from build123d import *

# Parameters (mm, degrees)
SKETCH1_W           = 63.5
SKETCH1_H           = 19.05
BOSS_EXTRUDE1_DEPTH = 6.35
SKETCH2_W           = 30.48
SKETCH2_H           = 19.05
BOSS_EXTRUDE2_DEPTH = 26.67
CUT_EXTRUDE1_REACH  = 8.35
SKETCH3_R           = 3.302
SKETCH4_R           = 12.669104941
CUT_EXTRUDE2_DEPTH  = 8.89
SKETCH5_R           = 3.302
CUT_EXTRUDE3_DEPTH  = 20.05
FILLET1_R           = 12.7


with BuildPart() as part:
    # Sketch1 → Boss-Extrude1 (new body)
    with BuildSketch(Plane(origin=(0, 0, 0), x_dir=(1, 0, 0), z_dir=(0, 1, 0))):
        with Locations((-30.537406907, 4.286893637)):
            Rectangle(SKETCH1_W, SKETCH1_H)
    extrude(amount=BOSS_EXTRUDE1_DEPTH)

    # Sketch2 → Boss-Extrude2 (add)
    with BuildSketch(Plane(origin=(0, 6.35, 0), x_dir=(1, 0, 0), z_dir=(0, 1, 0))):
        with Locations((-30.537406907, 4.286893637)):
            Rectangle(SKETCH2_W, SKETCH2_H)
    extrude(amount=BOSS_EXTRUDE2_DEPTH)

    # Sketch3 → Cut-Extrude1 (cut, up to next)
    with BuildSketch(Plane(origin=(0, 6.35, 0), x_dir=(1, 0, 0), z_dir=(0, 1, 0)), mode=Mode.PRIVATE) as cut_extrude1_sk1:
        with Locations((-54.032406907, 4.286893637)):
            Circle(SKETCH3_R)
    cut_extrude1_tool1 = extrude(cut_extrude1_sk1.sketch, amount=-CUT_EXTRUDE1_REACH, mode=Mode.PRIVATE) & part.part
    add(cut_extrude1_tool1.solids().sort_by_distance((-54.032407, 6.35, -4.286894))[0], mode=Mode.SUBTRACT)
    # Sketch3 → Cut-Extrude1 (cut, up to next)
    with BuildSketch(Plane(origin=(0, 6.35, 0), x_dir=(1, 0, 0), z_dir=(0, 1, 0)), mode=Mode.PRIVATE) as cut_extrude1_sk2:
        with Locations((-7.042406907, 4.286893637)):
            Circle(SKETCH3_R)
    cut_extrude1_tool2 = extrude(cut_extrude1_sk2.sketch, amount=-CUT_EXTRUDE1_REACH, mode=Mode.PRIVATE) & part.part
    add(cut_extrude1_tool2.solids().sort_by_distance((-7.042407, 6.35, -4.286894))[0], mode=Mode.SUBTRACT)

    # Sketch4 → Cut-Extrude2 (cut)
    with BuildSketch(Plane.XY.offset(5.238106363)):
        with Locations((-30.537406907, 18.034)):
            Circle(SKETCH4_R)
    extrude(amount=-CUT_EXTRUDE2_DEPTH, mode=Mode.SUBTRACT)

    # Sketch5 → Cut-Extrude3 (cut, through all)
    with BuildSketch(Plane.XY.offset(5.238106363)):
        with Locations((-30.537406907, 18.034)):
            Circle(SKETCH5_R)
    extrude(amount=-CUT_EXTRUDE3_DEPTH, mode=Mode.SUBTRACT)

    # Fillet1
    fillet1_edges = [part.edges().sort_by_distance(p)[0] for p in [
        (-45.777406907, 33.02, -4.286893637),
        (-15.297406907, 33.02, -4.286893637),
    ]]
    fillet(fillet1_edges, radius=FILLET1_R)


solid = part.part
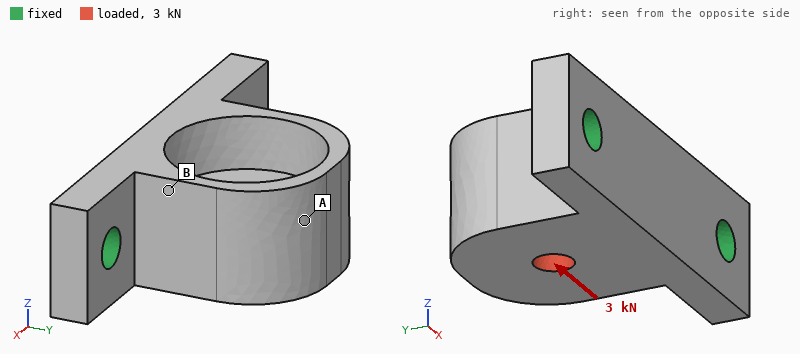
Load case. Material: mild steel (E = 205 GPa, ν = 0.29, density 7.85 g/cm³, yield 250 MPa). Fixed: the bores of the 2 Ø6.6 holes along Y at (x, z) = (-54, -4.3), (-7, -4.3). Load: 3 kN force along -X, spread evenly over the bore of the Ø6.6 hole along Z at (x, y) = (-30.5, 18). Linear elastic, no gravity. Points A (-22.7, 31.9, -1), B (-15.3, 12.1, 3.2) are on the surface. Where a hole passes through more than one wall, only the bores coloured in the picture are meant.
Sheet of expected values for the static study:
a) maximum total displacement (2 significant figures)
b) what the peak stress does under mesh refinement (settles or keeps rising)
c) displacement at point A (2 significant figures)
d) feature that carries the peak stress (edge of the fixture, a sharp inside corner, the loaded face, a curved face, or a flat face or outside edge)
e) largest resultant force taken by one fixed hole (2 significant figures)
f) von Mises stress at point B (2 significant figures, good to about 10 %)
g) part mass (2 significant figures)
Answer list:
8.1 µm
keeps rising
7.7 µm
edge of the fixture
1.9 kN
19 MPa
130 g
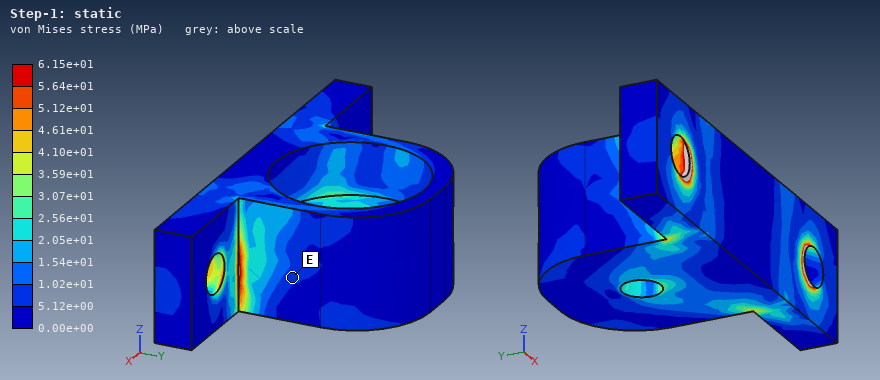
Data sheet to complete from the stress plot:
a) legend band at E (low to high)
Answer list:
5.12e+00 to 1.02e+01 MPa
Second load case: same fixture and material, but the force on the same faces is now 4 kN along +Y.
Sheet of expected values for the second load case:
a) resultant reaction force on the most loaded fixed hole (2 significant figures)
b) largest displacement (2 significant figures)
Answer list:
2.2 kN
22 µm
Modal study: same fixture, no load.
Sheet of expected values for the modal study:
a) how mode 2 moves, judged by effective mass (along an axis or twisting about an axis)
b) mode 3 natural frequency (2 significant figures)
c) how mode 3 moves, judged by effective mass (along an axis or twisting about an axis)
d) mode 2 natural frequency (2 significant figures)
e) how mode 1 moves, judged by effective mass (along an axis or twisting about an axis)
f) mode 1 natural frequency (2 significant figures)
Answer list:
along X
13 kHz
along Y
12 kHz
along Z
5000 Hz
